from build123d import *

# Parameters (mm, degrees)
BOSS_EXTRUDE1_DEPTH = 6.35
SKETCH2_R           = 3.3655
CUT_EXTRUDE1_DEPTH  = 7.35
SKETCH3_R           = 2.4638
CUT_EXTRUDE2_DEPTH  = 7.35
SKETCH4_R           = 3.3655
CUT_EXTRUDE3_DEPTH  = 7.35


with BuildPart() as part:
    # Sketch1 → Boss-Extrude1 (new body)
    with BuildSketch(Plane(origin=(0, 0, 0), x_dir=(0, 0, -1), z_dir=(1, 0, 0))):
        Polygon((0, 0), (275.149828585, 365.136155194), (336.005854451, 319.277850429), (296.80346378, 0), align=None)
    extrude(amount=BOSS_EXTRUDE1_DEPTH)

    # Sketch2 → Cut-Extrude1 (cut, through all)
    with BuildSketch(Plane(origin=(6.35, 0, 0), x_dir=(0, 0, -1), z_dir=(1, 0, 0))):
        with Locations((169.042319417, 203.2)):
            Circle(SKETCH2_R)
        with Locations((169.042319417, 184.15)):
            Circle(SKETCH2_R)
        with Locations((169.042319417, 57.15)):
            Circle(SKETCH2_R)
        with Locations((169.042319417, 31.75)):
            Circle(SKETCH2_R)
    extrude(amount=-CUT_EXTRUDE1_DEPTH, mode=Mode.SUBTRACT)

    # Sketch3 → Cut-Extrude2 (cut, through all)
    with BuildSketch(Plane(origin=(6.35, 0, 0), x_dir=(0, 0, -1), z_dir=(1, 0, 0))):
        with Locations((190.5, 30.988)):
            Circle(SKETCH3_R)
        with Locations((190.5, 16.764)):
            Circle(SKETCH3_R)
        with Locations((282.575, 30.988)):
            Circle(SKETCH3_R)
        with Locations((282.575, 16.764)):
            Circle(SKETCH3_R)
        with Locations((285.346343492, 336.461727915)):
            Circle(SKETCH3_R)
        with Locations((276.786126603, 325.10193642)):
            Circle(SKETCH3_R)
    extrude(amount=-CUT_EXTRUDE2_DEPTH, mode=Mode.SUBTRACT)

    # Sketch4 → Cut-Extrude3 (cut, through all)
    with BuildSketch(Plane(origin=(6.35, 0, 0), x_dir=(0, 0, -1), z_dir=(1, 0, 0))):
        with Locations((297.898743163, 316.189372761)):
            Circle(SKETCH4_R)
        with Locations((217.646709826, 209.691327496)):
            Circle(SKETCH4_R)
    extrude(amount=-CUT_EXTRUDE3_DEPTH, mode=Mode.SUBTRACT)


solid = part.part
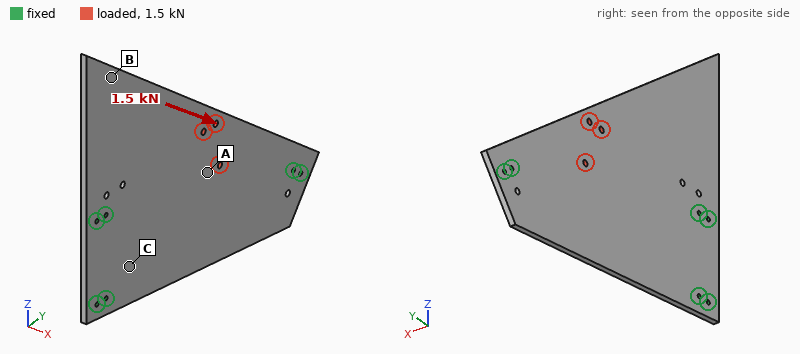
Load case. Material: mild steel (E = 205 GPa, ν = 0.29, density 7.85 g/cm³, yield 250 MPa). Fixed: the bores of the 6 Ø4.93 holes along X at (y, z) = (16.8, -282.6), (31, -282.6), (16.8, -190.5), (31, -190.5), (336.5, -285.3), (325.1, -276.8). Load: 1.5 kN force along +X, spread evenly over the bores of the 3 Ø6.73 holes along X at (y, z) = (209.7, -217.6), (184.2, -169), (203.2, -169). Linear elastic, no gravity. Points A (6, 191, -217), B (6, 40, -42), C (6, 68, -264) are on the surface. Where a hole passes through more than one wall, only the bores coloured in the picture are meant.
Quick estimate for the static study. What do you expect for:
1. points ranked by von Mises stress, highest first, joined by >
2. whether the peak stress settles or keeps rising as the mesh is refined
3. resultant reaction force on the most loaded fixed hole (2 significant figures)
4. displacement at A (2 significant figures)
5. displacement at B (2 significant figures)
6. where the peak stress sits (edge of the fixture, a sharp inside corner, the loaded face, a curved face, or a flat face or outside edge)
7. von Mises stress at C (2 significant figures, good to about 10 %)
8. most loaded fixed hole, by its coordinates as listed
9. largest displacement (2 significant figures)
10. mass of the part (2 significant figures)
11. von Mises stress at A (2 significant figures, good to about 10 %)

A > C > B
keeps rising
3.0 kN
0.55 mm
0.29 mm
edge of the fixture
32 MPa
(31, -190.5)
0.98 mm
3.2 kg
53 MPa
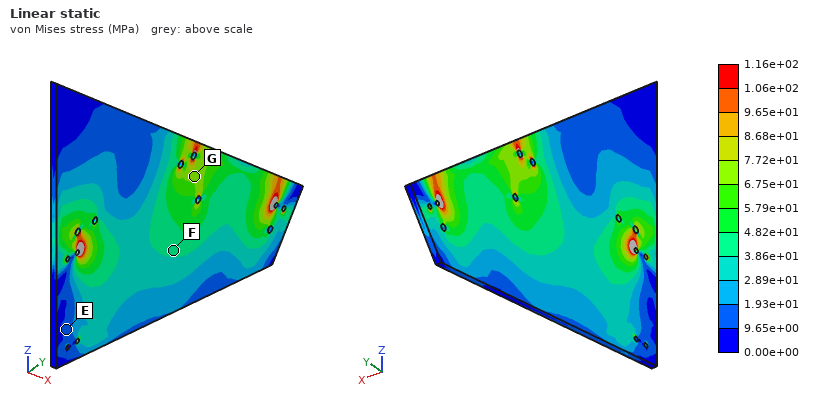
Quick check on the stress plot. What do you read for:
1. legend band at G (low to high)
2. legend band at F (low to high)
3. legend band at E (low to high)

6.75e+01 to 7.72e+01 MPa
3.86e+01 to 4.82e+01 MPa
9.65e+00 to 1.93e+01 MPa
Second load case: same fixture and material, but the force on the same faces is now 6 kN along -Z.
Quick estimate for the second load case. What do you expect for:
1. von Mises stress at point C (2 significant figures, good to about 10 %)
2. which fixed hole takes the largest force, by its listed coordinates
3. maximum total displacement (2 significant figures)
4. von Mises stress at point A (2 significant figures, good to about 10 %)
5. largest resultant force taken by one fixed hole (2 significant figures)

9.1 MPa
(325.1, -276.8)
15 µm
5.6 MPa
2.9 kN
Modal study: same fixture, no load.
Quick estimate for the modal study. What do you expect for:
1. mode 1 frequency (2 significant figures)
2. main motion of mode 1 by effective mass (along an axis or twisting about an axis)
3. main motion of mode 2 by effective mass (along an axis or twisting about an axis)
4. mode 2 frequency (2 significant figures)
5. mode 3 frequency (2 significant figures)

210 Hz
along X
along X
290 Hz
440 Hz
